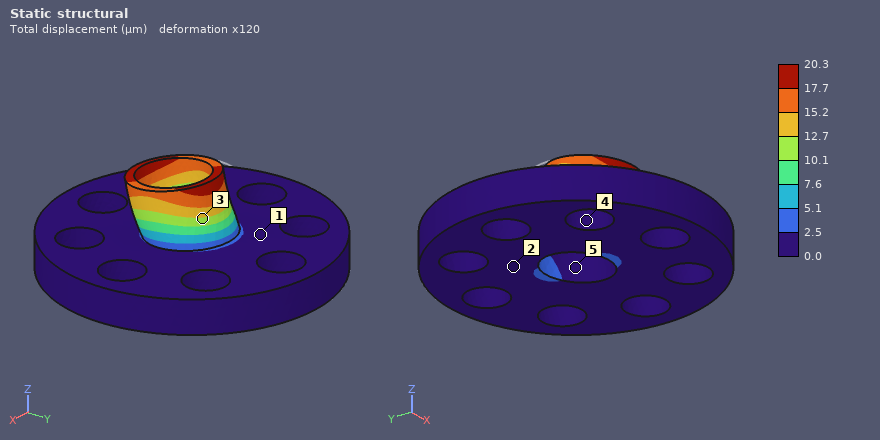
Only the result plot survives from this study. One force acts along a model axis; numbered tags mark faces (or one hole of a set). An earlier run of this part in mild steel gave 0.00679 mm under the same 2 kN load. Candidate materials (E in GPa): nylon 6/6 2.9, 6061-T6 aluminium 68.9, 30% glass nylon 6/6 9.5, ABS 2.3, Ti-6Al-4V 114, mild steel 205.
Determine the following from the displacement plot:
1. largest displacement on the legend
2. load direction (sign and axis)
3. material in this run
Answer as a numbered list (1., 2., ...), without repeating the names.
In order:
1. 20.3 µm
2. -Y
3. 6061-T6 aluminium
